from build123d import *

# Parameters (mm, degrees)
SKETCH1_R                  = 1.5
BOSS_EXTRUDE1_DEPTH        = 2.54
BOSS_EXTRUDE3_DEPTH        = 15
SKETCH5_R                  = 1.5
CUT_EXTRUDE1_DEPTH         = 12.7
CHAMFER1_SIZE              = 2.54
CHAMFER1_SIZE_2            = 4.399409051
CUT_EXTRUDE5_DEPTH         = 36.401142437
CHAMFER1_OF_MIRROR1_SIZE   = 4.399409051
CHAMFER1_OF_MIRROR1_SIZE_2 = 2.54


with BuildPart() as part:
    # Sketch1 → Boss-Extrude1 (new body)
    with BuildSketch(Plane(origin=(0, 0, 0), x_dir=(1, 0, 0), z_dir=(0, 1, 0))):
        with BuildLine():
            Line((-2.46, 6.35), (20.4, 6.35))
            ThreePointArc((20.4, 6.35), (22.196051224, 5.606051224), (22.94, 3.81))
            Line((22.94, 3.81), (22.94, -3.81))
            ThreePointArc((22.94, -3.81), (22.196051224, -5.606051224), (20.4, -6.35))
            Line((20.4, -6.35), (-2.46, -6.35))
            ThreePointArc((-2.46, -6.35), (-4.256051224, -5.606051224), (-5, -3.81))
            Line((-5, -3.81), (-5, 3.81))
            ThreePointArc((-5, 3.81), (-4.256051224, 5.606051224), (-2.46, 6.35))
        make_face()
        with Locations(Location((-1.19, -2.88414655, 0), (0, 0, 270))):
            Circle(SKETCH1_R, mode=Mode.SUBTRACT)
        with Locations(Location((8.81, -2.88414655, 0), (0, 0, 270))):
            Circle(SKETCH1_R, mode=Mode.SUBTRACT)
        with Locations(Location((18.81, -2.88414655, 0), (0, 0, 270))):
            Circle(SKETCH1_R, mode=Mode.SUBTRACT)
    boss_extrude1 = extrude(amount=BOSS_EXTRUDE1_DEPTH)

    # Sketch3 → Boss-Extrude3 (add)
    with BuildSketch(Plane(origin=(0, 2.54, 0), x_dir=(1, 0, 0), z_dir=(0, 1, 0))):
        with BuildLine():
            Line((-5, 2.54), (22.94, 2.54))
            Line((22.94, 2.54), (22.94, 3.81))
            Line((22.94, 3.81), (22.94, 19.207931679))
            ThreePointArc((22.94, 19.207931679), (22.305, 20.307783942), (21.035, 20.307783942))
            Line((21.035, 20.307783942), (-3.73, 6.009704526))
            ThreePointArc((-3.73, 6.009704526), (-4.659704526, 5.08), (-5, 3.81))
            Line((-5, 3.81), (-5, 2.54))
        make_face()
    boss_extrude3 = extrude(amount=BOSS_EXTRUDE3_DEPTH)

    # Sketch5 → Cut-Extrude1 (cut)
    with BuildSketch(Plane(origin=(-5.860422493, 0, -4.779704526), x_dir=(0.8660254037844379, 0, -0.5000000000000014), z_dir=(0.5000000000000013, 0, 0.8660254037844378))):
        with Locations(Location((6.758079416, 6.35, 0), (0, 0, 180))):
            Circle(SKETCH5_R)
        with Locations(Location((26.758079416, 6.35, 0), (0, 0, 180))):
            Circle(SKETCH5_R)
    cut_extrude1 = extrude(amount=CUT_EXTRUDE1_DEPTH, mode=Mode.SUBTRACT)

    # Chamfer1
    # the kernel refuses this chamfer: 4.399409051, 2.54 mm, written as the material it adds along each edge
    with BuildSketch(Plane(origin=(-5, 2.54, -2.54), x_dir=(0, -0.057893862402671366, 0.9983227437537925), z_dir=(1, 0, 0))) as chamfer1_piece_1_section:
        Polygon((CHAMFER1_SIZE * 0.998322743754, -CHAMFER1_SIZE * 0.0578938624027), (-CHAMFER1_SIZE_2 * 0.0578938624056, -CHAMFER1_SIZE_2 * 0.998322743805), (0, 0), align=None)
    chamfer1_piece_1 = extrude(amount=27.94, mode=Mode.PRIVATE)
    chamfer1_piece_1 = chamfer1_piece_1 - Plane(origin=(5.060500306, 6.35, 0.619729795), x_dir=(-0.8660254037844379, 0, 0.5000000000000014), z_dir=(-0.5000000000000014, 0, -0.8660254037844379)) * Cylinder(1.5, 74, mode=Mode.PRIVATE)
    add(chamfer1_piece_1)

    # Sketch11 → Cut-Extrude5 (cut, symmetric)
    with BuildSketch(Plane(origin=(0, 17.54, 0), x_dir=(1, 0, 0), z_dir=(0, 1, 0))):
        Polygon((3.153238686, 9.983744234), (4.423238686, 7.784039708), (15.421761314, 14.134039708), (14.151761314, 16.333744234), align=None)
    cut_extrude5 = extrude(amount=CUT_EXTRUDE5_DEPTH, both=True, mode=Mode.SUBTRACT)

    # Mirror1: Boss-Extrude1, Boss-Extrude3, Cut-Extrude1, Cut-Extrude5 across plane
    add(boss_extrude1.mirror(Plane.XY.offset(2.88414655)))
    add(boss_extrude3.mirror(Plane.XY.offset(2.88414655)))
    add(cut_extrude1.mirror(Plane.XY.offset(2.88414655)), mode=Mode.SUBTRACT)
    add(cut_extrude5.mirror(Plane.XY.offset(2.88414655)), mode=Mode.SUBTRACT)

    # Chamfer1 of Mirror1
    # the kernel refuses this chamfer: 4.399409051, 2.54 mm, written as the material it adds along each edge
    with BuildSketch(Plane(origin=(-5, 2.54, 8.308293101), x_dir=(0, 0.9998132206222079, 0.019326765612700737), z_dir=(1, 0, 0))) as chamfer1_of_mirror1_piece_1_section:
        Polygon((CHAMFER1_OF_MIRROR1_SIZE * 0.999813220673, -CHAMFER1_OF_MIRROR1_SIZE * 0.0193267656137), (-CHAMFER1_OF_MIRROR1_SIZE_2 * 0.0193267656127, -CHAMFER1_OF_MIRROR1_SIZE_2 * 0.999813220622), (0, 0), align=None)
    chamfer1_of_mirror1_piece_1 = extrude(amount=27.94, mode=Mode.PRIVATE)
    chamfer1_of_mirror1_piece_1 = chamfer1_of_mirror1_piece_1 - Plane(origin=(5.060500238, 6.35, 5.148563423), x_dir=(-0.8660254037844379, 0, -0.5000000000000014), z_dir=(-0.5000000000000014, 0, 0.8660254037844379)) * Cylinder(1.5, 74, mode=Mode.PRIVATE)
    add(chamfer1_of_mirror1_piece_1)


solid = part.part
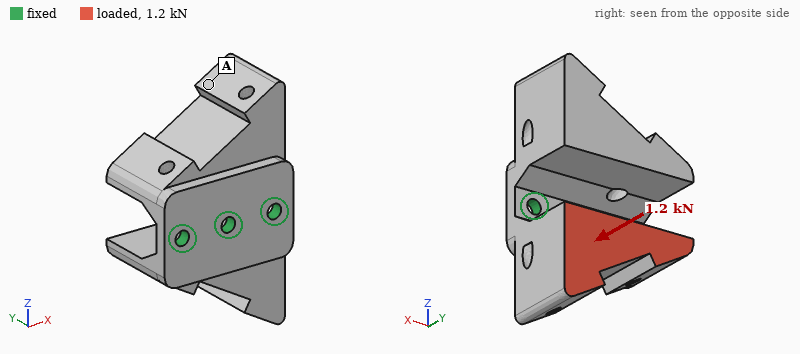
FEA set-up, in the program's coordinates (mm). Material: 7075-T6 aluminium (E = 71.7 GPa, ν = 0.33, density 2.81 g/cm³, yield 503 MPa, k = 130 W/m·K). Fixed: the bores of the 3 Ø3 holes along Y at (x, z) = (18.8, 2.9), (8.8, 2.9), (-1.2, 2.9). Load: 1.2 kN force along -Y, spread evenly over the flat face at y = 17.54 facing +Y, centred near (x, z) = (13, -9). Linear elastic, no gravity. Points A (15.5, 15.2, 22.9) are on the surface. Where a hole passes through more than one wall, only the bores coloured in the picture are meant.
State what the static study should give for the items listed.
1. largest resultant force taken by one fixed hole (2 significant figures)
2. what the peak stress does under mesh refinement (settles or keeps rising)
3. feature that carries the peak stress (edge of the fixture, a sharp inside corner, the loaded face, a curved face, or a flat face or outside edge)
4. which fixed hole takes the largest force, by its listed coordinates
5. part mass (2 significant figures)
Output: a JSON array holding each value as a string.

["620 N", "keeps rising", "edge of the fixture", "(18.8, 2.9)", "26 g"]
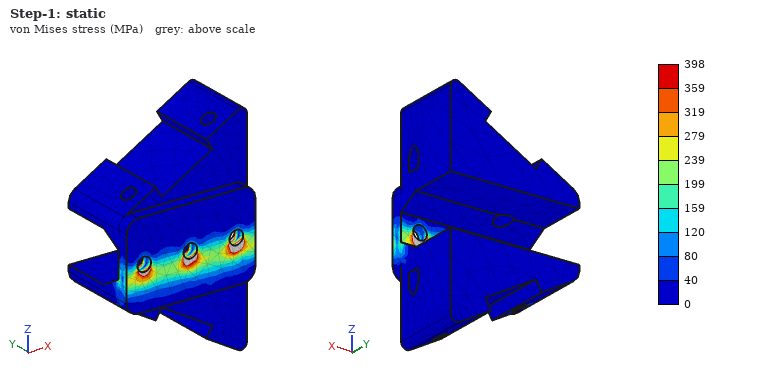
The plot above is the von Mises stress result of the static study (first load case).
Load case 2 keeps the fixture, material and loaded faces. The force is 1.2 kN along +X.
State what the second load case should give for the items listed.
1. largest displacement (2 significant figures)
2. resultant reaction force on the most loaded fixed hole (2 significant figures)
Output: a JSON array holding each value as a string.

["53 µm", "1.2 kN"]
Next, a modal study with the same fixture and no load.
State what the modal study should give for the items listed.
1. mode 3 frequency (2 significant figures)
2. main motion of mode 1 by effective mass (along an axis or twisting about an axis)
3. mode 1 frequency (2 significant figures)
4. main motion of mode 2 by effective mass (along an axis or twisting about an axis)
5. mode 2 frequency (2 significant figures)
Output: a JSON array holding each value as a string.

["11 kHz", "along Z", "2800 Hz", "along Y", "3000 Hz"]
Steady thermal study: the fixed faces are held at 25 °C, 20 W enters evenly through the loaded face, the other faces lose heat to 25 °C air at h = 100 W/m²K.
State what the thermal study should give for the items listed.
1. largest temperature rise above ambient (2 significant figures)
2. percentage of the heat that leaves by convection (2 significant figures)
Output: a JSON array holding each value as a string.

["22 K", "14 %"]
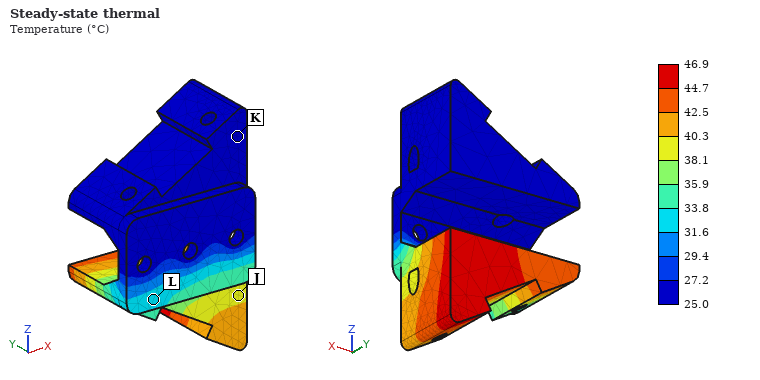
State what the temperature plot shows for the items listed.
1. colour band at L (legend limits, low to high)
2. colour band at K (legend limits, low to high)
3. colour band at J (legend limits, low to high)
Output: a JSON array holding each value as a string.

["31.6 to 33.8 °C", "25.0 to 27.2 °C", "38.1 to 40.3 °C"]
